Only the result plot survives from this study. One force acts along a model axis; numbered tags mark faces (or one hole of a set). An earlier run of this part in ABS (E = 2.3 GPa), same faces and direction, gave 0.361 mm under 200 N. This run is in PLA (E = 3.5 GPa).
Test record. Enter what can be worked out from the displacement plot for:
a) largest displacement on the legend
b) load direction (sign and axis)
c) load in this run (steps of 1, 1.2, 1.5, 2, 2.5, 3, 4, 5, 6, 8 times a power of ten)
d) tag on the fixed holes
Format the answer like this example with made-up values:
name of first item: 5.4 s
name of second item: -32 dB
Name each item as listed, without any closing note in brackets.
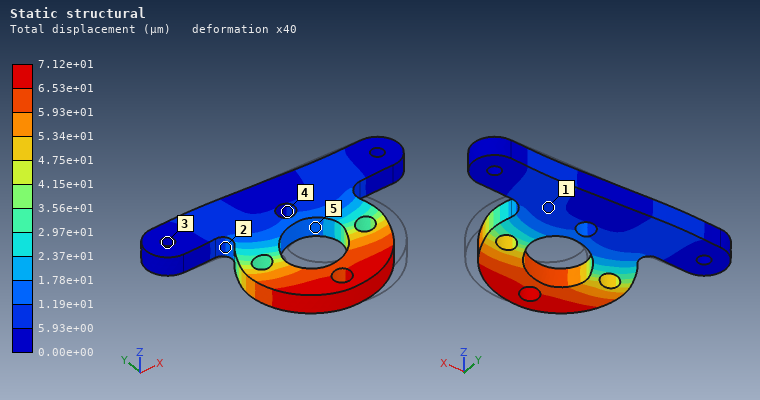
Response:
largest displacement on the legend: 7.12e+01 µm
load direction: -X
load in this run: 60 N
tag on the fixed holes: 3
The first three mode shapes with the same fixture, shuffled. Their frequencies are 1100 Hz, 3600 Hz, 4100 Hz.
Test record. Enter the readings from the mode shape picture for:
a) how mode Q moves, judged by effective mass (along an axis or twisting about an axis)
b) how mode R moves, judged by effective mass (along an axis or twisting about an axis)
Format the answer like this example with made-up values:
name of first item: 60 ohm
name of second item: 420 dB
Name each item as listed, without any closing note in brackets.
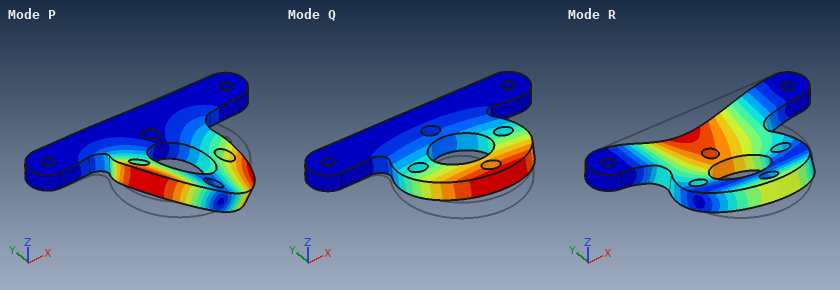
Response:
how mode Q moves, judged by effective mass: along Z
how mode R moves, judged by effective mass: along Z
